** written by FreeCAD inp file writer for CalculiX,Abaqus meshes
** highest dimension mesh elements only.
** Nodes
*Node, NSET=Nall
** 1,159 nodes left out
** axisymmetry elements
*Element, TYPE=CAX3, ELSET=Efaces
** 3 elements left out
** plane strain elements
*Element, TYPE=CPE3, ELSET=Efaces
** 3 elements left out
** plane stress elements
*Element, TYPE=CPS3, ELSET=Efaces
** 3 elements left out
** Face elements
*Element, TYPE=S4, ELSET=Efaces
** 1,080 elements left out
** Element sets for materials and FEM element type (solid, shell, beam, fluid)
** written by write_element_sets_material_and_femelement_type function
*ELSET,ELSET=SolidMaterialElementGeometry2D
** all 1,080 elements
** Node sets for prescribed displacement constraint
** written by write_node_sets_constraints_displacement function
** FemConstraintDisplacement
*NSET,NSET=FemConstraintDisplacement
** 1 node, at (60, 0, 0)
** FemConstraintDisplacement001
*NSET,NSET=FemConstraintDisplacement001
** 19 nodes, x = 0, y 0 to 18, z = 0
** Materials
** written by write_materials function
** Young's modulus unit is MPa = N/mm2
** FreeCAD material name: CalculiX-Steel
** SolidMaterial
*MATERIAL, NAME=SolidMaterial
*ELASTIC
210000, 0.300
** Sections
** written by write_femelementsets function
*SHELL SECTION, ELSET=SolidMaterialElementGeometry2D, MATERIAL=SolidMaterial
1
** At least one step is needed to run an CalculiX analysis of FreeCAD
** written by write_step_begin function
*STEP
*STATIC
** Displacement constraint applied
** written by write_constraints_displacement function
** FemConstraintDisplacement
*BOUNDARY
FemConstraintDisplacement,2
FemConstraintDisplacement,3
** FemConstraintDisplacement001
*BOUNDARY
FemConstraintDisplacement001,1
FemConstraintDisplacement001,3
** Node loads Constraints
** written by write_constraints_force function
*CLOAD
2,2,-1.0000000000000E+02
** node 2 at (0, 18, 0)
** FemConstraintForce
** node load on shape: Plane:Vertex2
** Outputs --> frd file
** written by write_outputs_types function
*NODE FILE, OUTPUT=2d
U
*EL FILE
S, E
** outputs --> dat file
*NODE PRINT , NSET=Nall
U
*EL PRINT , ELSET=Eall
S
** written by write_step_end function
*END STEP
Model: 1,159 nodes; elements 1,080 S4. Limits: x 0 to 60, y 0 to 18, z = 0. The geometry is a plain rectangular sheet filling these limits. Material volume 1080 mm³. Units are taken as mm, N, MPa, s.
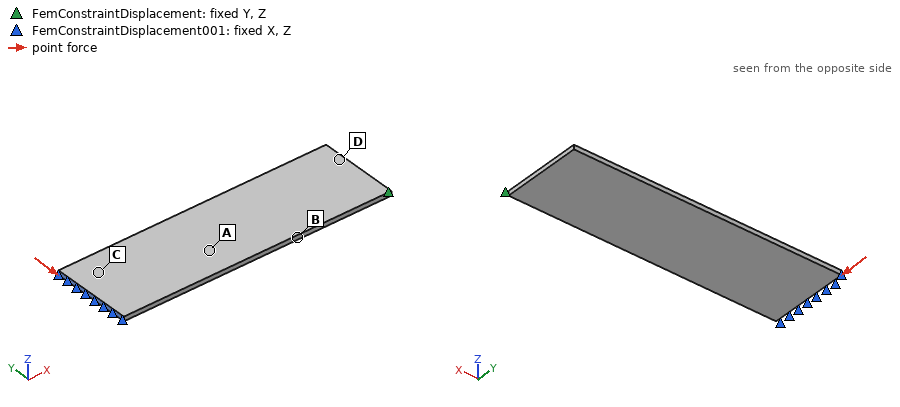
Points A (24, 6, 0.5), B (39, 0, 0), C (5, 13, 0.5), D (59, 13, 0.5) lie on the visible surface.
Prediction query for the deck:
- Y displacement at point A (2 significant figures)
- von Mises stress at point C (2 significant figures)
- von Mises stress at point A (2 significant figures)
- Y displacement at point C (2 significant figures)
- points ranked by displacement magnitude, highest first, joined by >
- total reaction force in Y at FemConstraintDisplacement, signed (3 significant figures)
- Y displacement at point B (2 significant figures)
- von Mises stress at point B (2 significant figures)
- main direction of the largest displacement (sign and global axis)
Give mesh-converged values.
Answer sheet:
-0.064 mm
46 MPa
26 MPa
-0.079 mm
C > A > B > D
100 N
-0.042 mm
39 MPa
-Y
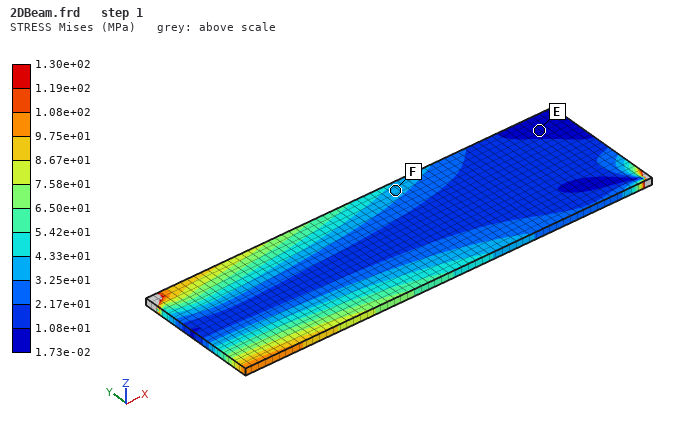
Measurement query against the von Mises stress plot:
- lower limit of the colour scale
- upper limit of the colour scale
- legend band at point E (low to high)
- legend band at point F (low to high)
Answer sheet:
1.73e-02 MPa
1.30e+02 MPa
1.73e-02 to 1.08e+01 MPa
3.25e+01 to 4.33e+01 MPa
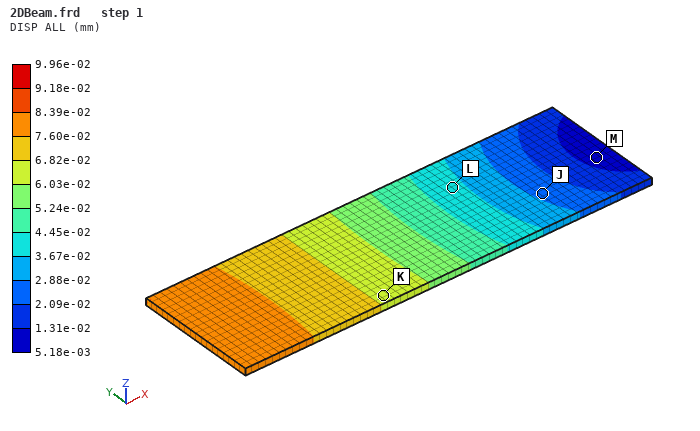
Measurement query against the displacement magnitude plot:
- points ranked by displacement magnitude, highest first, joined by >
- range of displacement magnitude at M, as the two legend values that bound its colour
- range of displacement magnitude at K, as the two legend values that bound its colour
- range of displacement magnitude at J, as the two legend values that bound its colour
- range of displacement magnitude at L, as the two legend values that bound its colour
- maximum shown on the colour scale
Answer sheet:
K > L > J > M
5.18e-03 to 1.31e-02 mm
6.03e-02 to 6.82e-02 mm
2.09e-02 to 2.88e-02 mm
3.67e-02 to 4.45e-02 mm
9.96e-02 mm
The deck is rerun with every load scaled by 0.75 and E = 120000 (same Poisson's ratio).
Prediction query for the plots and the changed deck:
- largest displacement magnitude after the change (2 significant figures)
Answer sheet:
0.13 mm
